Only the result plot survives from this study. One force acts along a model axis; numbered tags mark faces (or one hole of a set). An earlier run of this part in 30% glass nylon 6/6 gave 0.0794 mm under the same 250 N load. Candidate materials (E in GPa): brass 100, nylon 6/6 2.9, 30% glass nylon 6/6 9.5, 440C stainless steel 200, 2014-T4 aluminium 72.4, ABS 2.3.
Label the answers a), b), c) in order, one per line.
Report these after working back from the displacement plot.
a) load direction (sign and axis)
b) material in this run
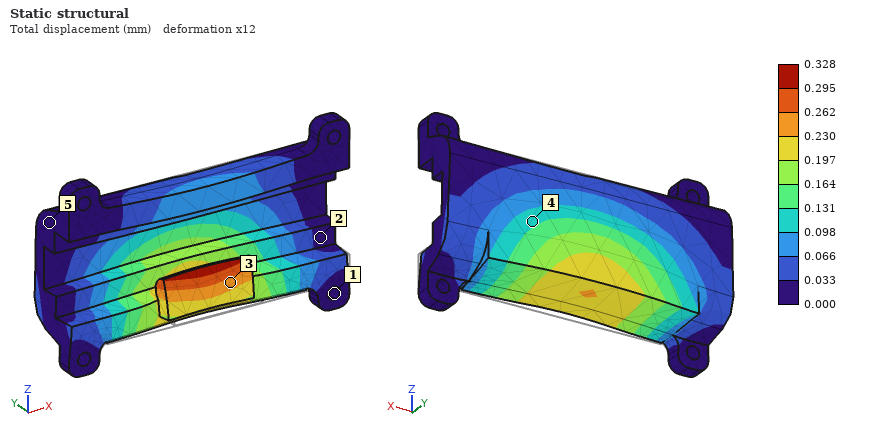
a) +Y
b) ABS
